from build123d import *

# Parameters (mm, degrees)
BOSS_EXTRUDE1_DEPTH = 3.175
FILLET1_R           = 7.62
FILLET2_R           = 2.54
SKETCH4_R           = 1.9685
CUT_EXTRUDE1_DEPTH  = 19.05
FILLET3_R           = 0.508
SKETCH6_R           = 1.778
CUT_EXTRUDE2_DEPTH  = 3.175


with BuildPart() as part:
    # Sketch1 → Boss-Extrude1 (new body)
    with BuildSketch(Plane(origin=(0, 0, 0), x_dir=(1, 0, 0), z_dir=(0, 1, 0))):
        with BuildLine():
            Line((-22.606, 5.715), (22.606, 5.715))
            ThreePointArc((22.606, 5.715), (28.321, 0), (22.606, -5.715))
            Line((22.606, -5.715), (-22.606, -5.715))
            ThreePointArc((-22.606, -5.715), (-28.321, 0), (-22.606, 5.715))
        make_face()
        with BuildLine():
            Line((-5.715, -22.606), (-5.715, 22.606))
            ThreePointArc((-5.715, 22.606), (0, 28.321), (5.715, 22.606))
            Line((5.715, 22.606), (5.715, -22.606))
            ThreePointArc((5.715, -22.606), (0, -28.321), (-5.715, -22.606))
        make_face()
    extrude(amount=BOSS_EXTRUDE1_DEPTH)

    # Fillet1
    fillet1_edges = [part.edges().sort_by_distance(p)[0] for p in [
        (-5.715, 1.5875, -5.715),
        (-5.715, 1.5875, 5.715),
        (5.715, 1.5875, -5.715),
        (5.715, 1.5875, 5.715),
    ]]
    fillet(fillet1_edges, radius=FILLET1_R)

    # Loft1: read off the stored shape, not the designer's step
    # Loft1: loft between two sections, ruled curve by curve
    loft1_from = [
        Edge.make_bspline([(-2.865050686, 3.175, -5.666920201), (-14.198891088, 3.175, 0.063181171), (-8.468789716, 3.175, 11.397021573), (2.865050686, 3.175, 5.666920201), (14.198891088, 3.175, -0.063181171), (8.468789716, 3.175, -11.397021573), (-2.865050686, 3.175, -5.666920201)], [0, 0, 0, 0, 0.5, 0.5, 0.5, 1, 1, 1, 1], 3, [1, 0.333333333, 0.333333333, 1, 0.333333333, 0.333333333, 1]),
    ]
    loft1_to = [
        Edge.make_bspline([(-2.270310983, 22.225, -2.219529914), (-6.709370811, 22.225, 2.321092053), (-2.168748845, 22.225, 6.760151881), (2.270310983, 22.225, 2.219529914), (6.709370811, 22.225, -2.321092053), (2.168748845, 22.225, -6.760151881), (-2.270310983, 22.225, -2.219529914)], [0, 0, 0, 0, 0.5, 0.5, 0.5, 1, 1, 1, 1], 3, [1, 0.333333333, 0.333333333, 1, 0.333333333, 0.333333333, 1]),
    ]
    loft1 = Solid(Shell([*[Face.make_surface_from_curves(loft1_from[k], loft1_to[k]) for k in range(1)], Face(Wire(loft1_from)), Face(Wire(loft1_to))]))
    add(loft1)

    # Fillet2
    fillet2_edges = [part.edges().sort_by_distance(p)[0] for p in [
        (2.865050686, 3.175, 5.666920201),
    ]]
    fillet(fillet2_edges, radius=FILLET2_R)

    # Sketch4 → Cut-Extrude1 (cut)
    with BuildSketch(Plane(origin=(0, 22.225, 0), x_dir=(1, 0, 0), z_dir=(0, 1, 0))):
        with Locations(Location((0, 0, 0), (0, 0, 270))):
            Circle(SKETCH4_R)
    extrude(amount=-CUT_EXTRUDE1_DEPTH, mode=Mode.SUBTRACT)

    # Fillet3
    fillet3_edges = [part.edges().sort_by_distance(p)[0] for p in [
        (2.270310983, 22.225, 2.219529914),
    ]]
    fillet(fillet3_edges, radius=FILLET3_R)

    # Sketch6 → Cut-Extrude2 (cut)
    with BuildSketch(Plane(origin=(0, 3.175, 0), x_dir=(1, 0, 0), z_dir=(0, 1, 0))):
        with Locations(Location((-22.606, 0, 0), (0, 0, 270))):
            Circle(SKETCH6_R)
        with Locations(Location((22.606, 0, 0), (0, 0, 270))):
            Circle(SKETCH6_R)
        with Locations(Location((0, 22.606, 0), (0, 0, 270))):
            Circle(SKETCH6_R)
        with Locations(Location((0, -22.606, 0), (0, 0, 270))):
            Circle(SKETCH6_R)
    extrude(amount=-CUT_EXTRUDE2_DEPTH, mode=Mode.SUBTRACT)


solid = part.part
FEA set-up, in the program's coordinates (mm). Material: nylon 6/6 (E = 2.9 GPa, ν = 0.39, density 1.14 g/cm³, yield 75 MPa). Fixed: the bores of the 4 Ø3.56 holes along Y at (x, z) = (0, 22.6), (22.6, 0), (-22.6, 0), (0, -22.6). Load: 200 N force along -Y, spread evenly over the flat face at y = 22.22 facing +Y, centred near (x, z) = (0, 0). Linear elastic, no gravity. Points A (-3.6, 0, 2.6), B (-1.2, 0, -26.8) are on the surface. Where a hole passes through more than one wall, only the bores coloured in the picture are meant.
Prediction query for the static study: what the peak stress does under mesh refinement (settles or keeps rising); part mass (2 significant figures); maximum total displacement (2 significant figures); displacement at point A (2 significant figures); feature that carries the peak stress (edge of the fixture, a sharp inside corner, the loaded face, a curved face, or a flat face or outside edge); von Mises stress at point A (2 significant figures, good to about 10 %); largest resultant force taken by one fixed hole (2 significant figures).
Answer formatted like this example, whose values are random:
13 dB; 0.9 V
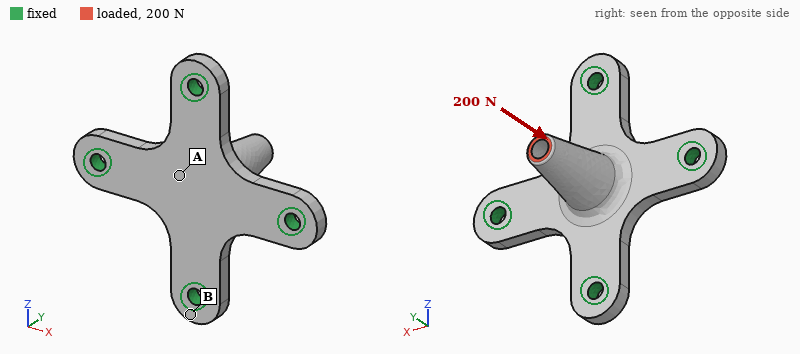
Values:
keeps rising; 5.4 g; 0.23 mm; 0.20 mm; edge of the fixture; 7.0 MPa; 52 N
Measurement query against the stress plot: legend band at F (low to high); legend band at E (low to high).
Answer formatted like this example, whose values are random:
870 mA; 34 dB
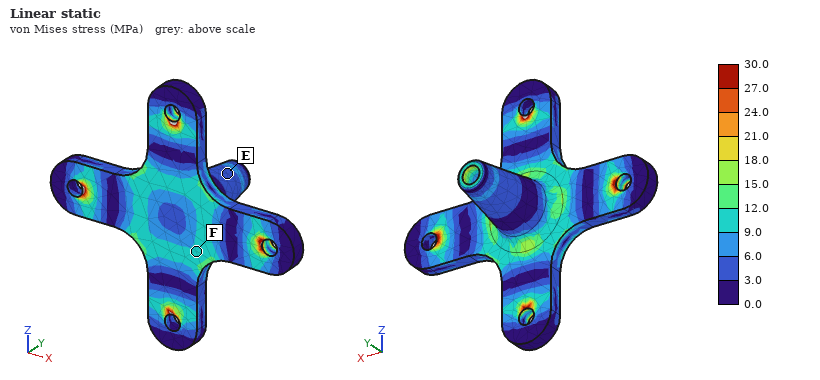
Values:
9.0 to 12.0 MPa; 3.0 to 6.0 MPa
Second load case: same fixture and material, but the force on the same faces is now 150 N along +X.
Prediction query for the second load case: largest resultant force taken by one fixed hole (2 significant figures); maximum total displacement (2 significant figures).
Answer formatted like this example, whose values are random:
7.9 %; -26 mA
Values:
110 N; 0.81 mm
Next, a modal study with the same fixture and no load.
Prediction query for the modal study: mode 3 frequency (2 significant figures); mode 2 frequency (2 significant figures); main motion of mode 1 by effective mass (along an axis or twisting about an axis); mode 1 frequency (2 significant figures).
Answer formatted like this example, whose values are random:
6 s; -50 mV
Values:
3800 Hz; 3800 Hz; along Y; 2900 Hz
